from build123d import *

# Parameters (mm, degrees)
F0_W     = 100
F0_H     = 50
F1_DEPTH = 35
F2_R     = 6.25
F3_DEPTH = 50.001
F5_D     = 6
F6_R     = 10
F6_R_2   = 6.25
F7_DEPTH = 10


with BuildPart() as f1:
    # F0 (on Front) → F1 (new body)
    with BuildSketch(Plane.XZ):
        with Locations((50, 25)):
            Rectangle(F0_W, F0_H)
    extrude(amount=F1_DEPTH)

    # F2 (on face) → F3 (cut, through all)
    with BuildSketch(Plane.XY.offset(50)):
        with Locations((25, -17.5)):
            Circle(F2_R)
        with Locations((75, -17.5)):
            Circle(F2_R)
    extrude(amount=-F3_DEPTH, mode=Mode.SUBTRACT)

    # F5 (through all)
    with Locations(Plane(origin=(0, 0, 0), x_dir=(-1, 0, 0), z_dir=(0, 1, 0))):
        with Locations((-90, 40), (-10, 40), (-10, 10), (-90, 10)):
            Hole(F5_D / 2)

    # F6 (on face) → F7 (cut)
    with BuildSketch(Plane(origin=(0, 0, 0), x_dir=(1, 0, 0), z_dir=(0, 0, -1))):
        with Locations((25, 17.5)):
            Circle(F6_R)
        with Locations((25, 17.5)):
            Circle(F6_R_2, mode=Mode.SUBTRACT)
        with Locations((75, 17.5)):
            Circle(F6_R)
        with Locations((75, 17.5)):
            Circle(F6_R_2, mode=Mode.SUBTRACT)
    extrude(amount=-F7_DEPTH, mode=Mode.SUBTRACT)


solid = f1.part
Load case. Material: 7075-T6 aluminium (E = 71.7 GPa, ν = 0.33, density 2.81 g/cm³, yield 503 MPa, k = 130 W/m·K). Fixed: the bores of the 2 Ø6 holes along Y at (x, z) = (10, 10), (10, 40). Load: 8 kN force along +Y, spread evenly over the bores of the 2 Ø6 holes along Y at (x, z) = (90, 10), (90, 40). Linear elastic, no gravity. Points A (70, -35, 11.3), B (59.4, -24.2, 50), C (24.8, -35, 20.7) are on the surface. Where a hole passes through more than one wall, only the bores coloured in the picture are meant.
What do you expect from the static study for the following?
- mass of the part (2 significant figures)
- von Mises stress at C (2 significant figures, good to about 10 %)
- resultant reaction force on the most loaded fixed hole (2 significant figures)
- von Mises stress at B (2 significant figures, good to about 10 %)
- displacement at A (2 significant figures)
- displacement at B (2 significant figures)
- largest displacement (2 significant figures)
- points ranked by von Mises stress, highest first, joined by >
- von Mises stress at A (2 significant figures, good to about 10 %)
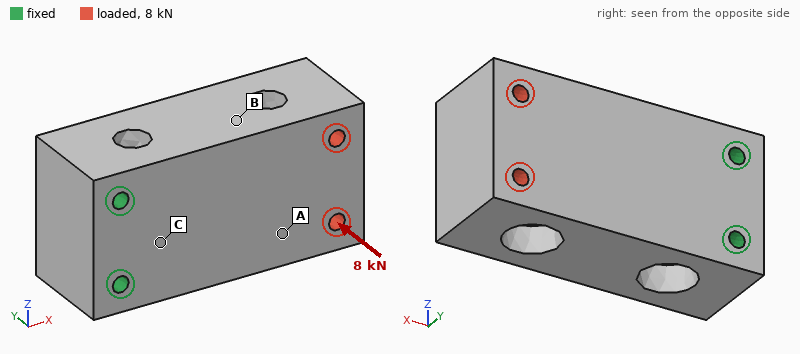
440 g
43 MPa
4.1 kN
13 MPa
0.11 mm
0.071 mm
0.18 mm
C > A > B
26 MPa
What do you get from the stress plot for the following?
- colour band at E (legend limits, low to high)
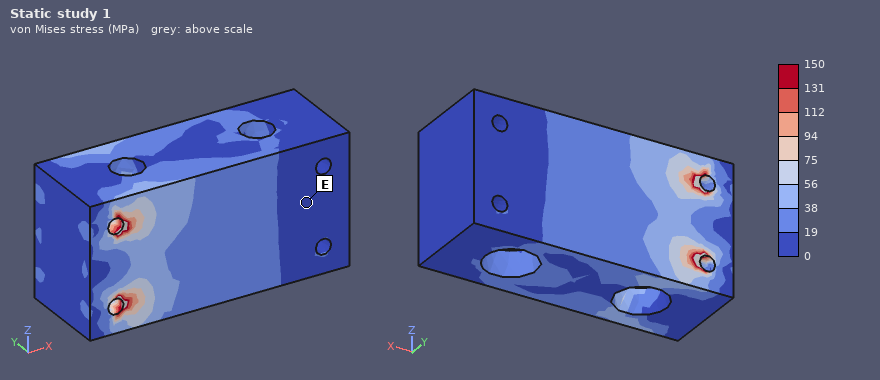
0 to 19 MPa
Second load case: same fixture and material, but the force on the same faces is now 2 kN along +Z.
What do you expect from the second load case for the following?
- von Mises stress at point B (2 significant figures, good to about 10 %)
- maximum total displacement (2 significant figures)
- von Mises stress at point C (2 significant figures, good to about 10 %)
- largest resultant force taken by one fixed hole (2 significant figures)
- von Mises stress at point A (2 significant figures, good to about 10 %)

4.3 MPa
31 µm
4.8 MPa
4.9 kN
3.1 MPa
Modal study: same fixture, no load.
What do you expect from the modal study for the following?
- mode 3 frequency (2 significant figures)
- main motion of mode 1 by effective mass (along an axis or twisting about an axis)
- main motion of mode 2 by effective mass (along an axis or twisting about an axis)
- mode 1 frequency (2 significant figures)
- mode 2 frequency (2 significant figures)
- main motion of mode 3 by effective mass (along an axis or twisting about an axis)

7000 Hz
along Y
along Z
3000 Hz
3600 Hz
twisting about X
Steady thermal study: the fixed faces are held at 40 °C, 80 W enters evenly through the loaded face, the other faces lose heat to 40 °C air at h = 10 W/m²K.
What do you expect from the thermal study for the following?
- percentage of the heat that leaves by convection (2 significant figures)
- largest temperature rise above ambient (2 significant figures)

5.2 %
37 K
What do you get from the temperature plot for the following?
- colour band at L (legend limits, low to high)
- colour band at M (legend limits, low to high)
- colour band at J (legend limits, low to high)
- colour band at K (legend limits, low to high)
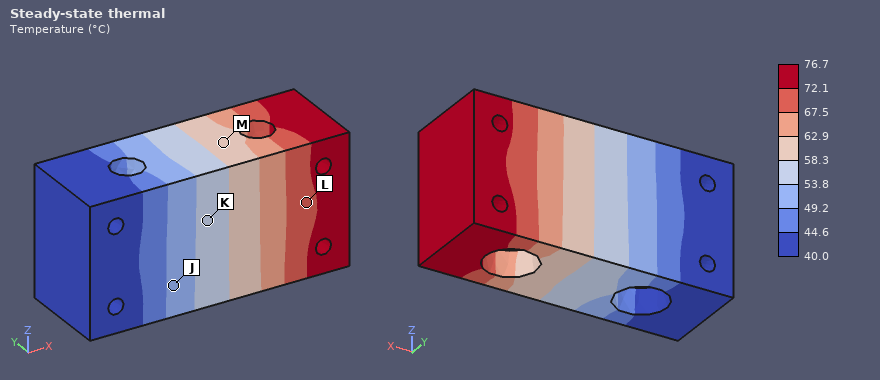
67.5 to 72.1 °C
58.3 to 62.9 °C
49.2 to 53.8 °C
53.8 to 58.3 °C
